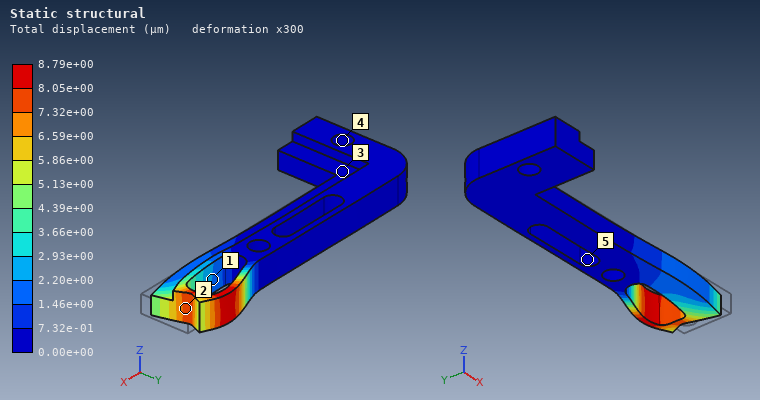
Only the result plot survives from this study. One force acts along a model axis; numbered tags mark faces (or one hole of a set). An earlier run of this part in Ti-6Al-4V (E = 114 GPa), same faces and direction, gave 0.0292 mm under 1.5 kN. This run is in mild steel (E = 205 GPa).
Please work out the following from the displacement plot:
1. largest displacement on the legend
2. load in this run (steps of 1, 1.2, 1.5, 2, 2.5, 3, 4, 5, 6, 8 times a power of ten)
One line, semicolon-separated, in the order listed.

8.79e+00 µm; 800 N
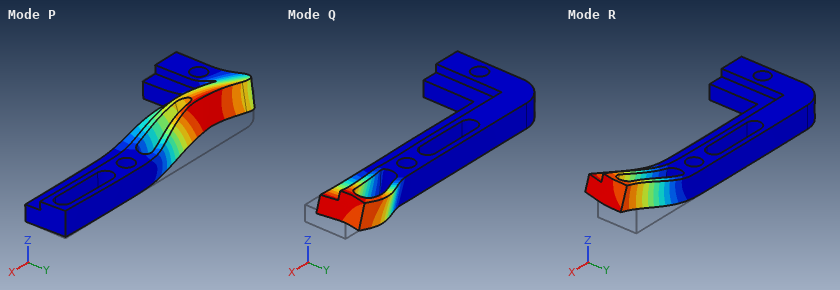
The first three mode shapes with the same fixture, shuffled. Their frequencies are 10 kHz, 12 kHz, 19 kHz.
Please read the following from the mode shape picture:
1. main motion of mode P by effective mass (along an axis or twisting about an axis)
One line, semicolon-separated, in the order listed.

along Z
